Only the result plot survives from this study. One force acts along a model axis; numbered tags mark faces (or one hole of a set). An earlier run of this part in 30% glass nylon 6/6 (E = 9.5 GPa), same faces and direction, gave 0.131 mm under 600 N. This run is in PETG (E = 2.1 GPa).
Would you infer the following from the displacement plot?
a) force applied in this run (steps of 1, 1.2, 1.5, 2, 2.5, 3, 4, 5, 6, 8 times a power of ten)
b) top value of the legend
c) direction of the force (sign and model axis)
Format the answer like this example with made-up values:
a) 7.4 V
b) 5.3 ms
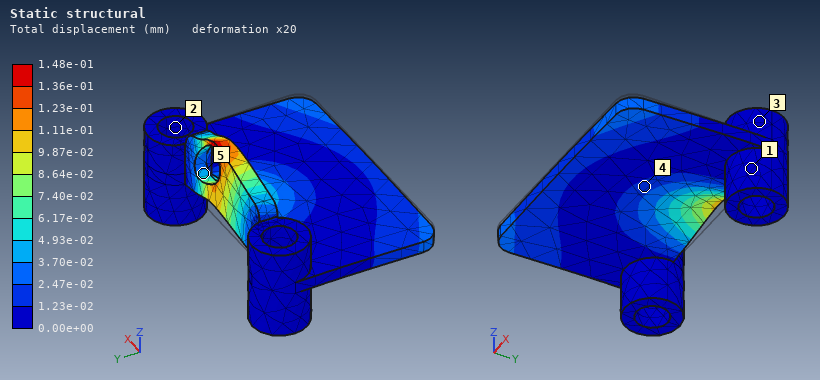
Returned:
a) 150 N
b) 1.48e-01 mm
c) +Z
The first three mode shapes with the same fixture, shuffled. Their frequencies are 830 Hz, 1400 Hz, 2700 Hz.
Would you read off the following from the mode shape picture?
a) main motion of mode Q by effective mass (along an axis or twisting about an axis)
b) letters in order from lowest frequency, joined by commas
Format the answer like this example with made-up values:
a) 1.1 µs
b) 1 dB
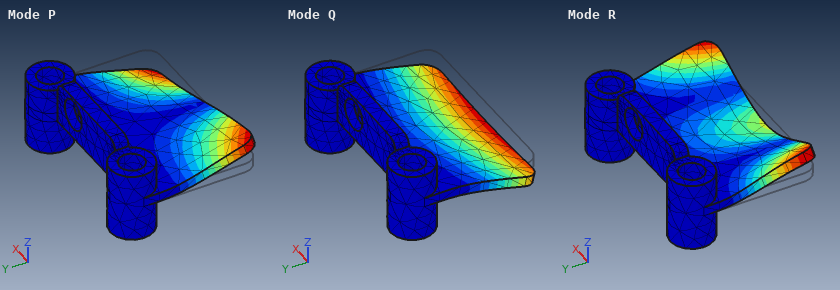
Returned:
a) along Z
b) Q, P, R
